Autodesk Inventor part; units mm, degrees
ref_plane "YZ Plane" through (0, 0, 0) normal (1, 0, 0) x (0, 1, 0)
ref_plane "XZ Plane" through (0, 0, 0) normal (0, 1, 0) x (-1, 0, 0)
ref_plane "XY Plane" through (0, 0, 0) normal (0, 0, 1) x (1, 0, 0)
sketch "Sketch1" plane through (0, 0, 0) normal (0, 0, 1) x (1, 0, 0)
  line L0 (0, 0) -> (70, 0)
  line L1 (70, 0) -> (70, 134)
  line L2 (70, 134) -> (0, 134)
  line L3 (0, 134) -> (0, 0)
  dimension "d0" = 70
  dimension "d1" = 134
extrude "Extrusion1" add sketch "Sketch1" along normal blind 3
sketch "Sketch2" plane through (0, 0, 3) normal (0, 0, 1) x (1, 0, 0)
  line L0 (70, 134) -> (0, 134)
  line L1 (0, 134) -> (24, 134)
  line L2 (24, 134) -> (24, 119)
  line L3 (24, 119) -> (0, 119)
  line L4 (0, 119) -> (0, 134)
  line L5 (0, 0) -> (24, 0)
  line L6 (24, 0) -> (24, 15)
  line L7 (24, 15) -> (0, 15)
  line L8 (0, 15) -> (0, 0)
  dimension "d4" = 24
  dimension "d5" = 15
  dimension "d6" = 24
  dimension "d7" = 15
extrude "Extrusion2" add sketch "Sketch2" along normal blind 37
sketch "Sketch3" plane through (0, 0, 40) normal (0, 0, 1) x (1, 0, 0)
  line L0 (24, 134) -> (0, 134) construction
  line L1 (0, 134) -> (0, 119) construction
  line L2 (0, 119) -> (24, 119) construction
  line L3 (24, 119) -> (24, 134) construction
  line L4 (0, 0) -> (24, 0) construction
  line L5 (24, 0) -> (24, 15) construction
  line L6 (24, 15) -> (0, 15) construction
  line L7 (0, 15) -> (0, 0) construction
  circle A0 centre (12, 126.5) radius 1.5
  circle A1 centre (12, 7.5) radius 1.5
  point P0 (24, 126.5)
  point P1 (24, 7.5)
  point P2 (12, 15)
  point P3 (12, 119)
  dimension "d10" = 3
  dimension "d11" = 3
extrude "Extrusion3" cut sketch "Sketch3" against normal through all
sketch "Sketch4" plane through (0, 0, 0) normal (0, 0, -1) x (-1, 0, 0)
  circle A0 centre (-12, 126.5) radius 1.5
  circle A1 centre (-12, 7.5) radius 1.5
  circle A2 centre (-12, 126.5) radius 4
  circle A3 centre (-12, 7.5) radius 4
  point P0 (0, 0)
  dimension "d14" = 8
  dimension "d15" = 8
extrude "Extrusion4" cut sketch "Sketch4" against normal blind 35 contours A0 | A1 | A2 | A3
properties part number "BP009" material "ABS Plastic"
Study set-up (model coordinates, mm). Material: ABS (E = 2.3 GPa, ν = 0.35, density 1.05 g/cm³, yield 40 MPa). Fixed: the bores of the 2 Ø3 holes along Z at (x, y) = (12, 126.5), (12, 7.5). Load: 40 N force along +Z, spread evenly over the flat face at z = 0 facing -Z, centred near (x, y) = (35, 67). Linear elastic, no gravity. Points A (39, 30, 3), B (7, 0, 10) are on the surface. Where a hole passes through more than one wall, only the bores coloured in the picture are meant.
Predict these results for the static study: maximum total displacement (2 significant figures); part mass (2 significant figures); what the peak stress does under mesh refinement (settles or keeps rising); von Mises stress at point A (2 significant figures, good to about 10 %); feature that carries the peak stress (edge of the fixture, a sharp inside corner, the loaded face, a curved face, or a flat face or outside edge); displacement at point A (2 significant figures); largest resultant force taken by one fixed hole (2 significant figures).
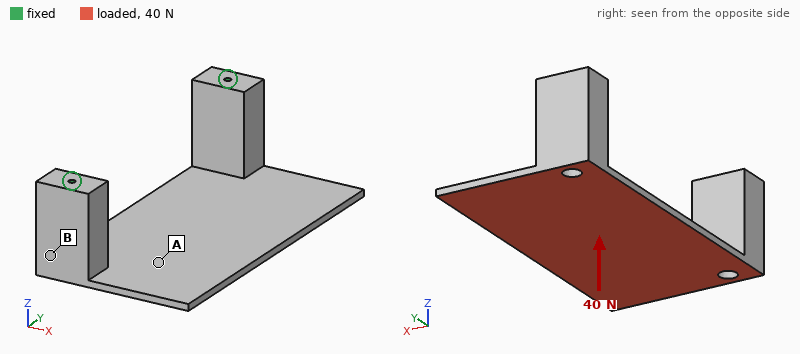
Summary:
1.6 mm
54 g
keeps rising
1.5 MPa
edge of the fixture
0.52 mm
22 N
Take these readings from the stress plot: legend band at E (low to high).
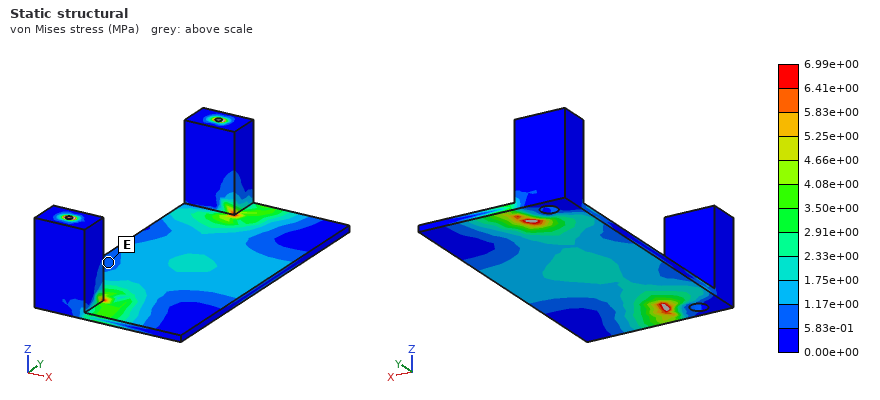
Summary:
5.83e-01 to 1.17e+00 MPa
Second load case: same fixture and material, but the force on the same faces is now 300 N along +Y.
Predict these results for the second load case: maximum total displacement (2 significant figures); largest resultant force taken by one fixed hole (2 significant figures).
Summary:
1.8 mm
160 N
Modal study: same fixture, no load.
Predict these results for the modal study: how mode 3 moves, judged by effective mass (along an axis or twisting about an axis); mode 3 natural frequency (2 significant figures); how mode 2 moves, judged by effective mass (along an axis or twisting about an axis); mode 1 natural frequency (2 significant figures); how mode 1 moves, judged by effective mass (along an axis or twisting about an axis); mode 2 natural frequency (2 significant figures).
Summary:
along X
390 Hz
along Y
190 Hz
along Z
330 Hz
